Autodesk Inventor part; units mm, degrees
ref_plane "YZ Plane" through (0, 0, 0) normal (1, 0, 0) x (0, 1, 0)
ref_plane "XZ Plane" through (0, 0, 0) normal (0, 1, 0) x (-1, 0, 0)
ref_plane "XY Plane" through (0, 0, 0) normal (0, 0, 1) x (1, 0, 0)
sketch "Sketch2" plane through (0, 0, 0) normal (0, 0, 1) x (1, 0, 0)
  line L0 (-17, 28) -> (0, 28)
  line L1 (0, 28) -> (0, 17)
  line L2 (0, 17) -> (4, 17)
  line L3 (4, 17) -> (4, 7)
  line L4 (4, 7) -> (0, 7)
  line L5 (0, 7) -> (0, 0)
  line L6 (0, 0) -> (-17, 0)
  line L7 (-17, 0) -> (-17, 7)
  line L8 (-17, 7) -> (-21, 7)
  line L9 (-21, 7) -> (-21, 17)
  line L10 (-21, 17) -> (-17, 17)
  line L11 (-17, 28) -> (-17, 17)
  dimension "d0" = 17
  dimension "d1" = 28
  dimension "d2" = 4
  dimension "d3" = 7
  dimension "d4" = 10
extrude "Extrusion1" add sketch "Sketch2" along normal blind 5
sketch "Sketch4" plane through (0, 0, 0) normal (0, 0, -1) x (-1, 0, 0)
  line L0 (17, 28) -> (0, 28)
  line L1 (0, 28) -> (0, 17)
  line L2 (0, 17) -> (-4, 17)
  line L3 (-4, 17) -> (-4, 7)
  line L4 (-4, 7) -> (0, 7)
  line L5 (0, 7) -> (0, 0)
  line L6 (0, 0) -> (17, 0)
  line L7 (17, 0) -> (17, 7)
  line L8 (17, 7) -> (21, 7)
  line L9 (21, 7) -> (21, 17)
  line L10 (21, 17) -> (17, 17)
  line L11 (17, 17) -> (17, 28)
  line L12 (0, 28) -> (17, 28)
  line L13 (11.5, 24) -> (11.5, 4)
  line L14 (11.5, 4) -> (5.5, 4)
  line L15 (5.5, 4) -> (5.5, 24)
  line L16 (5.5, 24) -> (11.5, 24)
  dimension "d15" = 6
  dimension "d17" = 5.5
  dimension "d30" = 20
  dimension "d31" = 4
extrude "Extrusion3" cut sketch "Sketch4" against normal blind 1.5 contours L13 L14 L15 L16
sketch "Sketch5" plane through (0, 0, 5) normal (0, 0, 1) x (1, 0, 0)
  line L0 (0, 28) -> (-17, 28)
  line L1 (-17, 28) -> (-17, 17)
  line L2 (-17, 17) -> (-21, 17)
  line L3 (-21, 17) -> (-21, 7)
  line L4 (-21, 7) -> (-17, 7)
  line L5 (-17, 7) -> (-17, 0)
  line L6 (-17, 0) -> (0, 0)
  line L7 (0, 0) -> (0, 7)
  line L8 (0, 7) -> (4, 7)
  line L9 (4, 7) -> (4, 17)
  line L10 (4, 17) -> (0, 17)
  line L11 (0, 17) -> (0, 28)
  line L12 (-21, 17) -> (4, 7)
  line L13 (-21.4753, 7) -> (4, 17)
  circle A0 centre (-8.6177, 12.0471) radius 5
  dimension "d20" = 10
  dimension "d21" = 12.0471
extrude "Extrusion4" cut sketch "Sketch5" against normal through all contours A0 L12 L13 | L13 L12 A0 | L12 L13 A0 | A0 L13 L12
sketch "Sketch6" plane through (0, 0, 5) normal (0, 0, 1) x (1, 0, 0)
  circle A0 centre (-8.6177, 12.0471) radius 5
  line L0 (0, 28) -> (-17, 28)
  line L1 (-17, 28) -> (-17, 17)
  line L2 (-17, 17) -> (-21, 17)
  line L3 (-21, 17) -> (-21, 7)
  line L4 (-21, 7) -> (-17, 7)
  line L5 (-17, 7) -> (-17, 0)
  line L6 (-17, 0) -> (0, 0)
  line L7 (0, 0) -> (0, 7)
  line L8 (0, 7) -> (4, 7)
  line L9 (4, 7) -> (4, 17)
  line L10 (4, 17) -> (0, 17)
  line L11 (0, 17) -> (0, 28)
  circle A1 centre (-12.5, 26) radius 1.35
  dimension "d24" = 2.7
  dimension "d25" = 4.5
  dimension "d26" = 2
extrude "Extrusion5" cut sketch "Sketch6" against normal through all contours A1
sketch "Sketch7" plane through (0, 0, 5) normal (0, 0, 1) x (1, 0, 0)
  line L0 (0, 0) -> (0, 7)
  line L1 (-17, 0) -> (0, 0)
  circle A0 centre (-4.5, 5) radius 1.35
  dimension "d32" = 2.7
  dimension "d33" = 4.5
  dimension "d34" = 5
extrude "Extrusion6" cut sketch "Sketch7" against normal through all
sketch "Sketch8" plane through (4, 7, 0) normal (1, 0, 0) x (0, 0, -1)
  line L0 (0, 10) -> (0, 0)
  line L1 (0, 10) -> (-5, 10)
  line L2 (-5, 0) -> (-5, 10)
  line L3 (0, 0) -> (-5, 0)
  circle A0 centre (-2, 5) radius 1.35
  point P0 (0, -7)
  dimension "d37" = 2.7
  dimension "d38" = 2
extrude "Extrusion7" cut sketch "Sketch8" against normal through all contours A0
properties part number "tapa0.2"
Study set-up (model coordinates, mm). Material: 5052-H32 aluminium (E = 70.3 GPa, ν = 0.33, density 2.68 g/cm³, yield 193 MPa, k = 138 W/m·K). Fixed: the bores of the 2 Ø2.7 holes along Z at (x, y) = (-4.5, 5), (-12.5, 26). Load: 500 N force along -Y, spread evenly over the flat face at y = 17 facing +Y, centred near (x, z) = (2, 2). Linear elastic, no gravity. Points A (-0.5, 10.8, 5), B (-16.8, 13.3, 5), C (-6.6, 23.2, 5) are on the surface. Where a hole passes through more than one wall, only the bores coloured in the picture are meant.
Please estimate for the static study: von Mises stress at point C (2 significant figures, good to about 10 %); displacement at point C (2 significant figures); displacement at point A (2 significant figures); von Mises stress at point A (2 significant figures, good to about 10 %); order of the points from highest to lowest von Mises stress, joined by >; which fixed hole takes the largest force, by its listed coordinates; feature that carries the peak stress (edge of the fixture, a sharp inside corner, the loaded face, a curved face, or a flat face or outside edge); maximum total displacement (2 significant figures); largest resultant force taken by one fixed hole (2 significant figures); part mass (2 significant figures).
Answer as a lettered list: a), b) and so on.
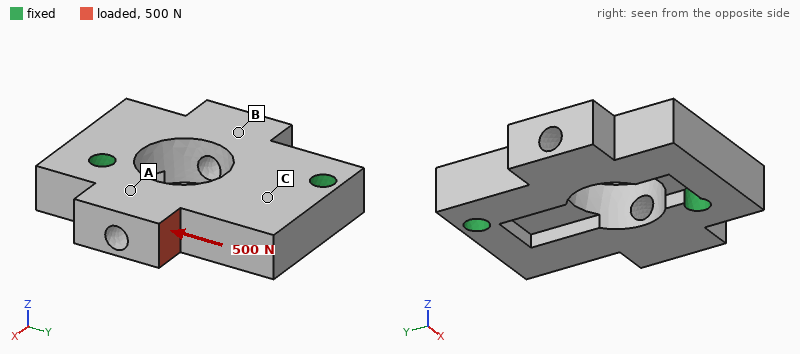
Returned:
a) 7.6 MPa
b) 1.1 µm
c) 2.0 µm
d) 19 MPa
e) A > C > B
f) (-4.5, 5)
g) a curved face
h) 6.4 µm
i) 390 N
j) 5.8 g
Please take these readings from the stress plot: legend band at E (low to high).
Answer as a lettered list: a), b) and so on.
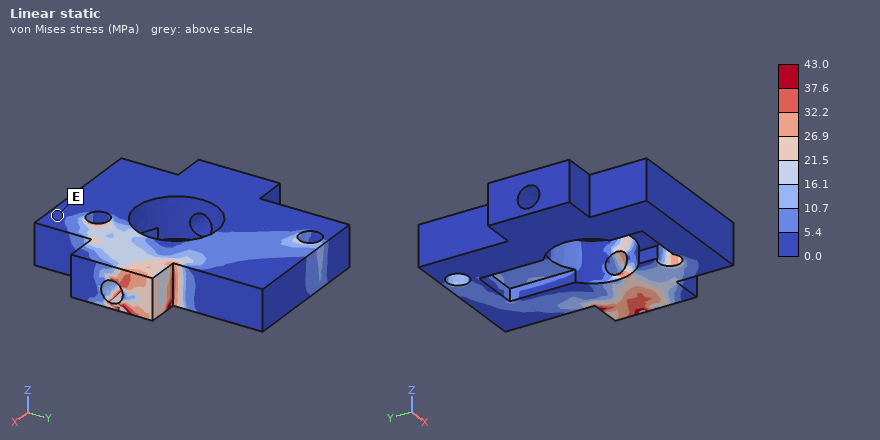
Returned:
a) 0.0 to 5.4 MPa
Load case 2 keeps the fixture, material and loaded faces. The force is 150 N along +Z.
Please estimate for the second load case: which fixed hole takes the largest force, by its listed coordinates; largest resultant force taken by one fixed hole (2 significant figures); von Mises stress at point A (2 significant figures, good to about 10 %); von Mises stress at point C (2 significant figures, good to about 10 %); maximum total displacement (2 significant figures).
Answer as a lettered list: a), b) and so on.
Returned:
a) (-4.5, 5)
b) 92 N
c) 21 MPa
d) 11 MPa
e) 17 µm
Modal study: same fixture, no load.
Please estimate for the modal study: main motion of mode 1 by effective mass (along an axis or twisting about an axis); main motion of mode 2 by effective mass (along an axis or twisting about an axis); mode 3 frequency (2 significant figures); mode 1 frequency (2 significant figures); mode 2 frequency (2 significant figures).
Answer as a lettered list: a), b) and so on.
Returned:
a) along Z
b) along Z
c) 35 kHz
d) 16 kHz
e) 22 kHz
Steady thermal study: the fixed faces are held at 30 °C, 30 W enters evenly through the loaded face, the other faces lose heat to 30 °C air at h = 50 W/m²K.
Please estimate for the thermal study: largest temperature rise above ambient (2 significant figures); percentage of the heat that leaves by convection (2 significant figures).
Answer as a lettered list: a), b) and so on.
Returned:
a) 75 K
b) 3.4 %
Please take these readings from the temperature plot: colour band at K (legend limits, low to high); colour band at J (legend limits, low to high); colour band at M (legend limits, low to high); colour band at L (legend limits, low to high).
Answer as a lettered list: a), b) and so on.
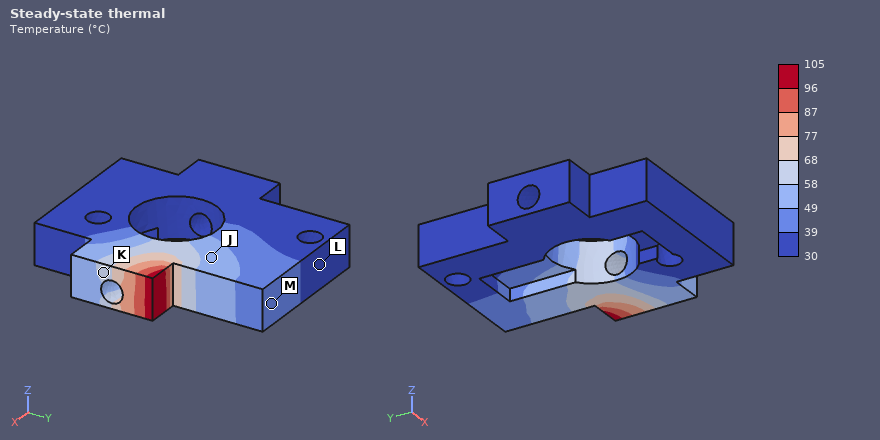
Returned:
a) 58 to 68 °C
b) 49 to 58 °C
c) 39 to 49 °C
d) 30 to 39 °C
